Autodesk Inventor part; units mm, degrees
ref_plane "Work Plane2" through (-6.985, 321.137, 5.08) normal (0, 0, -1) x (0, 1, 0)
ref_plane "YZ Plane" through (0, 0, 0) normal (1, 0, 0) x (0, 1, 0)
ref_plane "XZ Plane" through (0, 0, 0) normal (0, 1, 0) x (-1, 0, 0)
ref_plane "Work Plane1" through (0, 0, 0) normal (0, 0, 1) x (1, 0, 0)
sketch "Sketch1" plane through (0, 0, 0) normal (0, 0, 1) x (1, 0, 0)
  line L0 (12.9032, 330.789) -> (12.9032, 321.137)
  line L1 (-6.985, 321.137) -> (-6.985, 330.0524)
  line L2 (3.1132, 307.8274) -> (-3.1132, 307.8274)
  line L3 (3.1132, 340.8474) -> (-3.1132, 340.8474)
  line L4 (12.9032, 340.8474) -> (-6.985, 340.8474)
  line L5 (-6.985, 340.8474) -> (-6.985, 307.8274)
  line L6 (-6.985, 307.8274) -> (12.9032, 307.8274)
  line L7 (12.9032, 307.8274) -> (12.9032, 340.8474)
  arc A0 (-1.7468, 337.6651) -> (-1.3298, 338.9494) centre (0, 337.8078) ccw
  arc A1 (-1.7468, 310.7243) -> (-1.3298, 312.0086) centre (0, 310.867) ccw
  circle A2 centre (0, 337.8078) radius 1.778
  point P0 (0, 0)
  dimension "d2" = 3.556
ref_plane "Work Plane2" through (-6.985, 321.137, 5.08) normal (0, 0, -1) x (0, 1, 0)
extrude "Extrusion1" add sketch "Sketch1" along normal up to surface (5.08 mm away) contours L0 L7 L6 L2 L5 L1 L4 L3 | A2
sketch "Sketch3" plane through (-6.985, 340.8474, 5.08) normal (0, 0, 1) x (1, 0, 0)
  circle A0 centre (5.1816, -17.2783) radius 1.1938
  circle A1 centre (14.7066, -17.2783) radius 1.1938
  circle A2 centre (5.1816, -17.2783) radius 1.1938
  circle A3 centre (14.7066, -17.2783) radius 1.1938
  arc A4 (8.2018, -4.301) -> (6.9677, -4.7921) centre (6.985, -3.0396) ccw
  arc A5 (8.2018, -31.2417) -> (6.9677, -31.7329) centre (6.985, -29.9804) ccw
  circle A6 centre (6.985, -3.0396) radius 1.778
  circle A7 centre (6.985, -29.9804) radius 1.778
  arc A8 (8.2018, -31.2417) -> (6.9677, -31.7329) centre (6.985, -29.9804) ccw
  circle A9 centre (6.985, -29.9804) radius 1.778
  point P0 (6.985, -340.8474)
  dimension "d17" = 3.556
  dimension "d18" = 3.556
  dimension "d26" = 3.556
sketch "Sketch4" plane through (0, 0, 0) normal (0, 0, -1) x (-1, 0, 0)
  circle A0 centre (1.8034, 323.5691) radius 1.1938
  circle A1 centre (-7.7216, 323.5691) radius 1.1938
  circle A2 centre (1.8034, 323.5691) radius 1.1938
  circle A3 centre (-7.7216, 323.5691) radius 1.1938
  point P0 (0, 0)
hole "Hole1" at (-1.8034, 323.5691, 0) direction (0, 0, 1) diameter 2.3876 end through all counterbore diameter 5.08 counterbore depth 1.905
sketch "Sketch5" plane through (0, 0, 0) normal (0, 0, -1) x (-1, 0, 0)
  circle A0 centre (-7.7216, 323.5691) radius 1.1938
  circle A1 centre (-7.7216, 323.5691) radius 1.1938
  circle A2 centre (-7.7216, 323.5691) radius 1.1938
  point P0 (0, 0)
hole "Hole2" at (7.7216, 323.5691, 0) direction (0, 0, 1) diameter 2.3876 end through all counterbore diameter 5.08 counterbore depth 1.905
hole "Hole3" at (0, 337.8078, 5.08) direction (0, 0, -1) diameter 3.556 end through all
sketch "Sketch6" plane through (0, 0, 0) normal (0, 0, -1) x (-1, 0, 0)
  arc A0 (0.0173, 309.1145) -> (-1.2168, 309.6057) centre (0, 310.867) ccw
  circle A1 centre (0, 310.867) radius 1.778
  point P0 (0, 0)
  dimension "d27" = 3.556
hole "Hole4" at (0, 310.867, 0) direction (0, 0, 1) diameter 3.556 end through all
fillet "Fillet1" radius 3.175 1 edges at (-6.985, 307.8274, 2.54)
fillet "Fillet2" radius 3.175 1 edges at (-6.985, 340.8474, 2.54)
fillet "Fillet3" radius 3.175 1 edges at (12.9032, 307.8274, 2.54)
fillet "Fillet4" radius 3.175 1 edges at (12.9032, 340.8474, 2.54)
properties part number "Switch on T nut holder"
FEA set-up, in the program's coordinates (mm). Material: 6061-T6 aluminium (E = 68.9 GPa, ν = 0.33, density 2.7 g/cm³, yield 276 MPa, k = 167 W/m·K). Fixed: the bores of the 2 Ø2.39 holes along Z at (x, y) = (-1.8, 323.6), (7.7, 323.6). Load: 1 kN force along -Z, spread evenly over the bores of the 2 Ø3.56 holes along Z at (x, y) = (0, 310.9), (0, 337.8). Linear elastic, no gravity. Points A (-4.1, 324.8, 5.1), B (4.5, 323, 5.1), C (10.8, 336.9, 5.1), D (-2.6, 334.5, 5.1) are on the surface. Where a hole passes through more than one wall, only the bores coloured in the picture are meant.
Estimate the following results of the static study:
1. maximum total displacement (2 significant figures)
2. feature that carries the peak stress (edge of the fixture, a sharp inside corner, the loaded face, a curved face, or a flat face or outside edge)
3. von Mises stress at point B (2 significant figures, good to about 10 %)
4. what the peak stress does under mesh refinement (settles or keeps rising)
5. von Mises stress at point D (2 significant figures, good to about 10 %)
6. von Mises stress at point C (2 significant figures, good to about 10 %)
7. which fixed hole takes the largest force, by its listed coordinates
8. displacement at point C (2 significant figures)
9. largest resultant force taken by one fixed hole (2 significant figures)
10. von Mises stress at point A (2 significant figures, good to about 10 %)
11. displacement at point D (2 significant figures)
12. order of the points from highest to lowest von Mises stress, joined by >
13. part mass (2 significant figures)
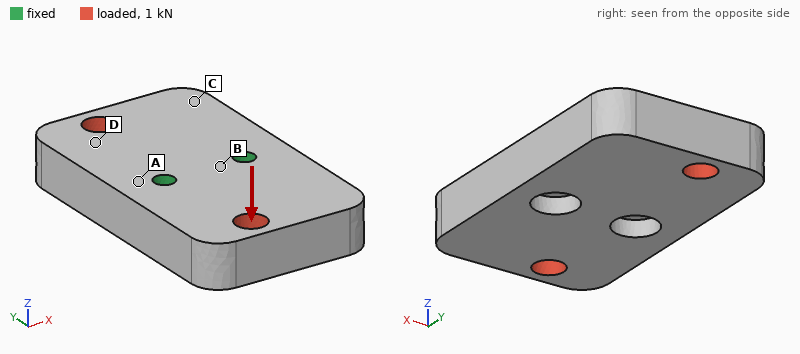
64 µm
edge of the fixture
72 MPa
keeps rising
32 MPa
13 MPa
(-1.8, 323.6)
32 µm
750 N
90 MPa
35 µm
A > B > D > C
8.3 g
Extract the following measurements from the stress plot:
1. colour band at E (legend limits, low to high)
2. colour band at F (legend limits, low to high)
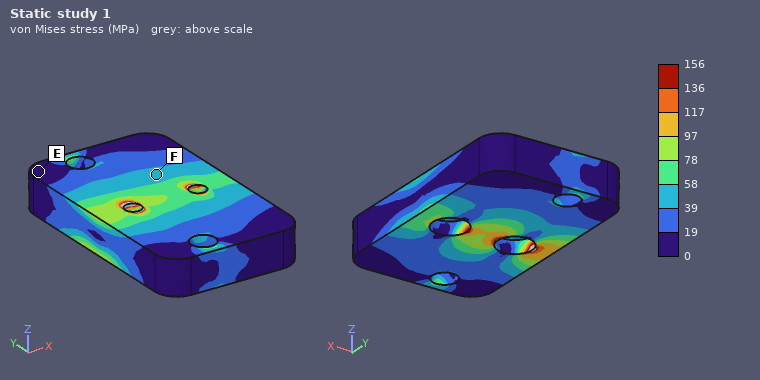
0 to 19 MPa
39 to 58 MPa
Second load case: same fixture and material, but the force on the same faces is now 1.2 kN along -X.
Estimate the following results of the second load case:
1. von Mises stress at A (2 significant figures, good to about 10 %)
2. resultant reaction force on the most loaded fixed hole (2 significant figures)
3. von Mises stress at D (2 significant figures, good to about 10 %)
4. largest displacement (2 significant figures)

22 MPa
620 N
11 MPa
9.6 µm
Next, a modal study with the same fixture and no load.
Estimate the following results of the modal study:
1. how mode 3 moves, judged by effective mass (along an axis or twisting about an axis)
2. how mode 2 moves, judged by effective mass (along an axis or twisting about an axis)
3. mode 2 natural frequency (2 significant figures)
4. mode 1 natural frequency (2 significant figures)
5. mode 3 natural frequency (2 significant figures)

twisting about Z
along Z
14 kHz
8800 Hz
21 kHz
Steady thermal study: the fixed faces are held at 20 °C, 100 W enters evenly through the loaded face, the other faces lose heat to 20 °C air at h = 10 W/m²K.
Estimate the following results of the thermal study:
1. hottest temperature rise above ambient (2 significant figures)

71 K
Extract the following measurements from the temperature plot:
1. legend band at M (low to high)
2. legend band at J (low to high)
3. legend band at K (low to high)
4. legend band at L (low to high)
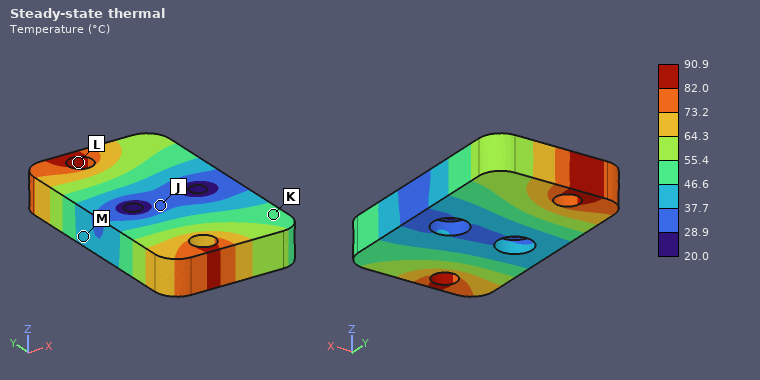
37.7 to 46.6 °C
28.9 to 37.7 °C
46.6 to 55.4 °C
82.0 to 90.9 °C
